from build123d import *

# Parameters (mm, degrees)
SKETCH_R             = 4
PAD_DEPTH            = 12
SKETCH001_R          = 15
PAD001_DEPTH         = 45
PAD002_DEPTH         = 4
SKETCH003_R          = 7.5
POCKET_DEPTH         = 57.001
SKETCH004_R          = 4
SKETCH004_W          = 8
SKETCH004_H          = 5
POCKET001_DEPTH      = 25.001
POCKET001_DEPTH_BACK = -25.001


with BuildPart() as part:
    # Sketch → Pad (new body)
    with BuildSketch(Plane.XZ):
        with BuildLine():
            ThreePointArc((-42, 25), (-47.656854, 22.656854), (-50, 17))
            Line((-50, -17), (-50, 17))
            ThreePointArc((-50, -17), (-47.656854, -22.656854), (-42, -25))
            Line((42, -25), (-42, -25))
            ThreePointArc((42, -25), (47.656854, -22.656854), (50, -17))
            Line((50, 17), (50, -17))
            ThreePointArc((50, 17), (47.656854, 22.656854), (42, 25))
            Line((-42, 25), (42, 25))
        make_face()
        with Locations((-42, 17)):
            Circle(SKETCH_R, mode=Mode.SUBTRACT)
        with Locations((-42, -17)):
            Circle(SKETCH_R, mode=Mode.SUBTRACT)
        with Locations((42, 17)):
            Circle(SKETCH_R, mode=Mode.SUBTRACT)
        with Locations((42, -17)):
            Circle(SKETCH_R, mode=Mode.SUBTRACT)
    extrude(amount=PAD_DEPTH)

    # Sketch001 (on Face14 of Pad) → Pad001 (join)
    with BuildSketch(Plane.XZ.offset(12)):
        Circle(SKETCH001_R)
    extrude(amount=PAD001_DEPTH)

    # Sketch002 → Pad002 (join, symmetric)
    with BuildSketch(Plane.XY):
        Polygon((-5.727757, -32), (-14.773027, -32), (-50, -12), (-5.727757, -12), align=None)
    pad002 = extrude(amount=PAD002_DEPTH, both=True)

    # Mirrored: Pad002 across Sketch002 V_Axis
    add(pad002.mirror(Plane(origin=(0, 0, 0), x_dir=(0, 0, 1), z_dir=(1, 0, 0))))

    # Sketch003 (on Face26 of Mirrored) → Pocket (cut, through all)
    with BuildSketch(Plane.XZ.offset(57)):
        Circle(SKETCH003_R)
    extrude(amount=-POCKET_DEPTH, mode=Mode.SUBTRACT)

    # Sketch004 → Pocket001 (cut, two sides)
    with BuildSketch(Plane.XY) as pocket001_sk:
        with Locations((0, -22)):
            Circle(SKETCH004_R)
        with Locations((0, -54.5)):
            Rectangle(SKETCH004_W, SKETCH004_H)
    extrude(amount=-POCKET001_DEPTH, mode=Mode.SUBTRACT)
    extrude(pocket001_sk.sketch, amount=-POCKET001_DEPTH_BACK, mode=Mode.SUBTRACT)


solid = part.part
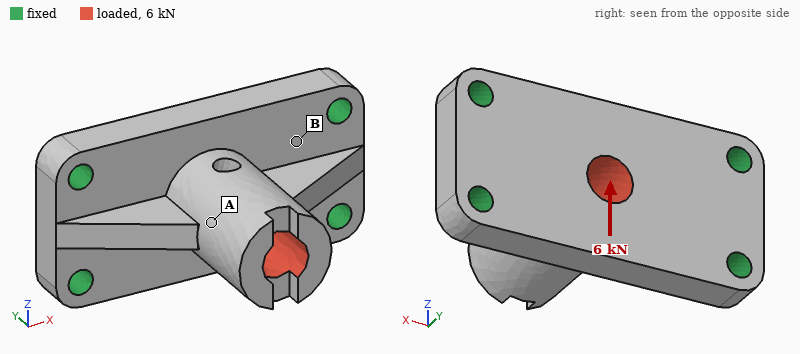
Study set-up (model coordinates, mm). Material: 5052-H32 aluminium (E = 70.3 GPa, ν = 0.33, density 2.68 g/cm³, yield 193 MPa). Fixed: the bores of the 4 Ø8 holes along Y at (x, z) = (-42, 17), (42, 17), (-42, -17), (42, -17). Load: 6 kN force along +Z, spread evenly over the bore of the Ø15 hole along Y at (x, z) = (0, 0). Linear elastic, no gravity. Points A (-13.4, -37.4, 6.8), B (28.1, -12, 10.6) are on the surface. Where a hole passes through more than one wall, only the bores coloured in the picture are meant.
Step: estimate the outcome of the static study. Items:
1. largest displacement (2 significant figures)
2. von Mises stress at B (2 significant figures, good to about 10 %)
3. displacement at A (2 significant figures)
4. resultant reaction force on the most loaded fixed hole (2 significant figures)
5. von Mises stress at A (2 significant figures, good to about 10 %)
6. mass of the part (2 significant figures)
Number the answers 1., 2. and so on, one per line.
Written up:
1. 0.13 mm
2. 34 MPa
3. 0.078 mm
4. 2.9 kN
5. 12 MPa
6. 220 g
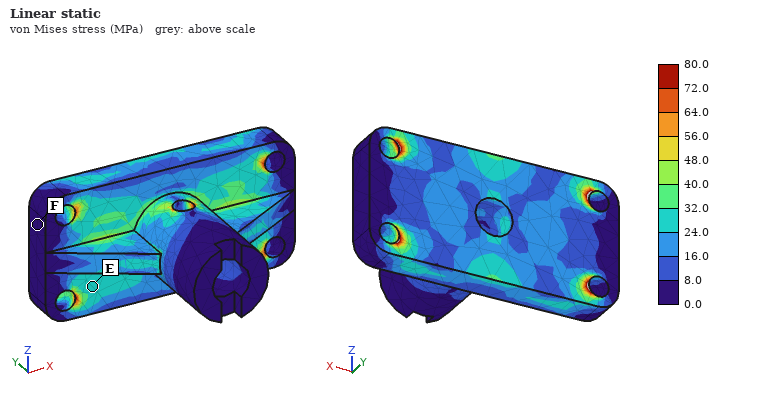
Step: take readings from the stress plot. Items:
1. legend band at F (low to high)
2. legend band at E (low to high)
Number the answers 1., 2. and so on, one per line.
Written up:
1. 0.0 to 8.0 MPa
2. 24.0 to 32.0 MPa
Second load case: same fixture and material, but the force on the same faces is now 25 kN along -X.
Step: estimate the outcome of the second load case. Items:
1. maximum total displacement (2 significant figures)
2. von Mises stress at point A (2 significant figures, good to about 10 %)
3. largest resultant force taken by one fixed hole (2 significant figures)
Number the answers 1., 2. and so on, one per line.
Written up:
1. 0.12 mm
2. 26 MPa
3. 7.5 kN
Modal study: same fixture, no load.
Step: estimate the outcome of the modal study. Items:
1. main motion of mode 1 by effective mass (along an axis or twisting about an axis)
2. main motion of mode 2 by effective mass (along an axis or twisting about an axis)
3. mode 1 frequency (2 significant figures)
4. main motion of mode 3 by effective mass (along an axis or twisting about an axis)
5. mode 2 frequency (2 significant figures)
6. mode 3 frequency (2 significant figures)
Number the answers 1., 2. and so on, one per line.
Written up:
1. along Z
2. along Y
3. 4400 Hz
4. along X
5. 7700 Hz
6. 9700 Hz
